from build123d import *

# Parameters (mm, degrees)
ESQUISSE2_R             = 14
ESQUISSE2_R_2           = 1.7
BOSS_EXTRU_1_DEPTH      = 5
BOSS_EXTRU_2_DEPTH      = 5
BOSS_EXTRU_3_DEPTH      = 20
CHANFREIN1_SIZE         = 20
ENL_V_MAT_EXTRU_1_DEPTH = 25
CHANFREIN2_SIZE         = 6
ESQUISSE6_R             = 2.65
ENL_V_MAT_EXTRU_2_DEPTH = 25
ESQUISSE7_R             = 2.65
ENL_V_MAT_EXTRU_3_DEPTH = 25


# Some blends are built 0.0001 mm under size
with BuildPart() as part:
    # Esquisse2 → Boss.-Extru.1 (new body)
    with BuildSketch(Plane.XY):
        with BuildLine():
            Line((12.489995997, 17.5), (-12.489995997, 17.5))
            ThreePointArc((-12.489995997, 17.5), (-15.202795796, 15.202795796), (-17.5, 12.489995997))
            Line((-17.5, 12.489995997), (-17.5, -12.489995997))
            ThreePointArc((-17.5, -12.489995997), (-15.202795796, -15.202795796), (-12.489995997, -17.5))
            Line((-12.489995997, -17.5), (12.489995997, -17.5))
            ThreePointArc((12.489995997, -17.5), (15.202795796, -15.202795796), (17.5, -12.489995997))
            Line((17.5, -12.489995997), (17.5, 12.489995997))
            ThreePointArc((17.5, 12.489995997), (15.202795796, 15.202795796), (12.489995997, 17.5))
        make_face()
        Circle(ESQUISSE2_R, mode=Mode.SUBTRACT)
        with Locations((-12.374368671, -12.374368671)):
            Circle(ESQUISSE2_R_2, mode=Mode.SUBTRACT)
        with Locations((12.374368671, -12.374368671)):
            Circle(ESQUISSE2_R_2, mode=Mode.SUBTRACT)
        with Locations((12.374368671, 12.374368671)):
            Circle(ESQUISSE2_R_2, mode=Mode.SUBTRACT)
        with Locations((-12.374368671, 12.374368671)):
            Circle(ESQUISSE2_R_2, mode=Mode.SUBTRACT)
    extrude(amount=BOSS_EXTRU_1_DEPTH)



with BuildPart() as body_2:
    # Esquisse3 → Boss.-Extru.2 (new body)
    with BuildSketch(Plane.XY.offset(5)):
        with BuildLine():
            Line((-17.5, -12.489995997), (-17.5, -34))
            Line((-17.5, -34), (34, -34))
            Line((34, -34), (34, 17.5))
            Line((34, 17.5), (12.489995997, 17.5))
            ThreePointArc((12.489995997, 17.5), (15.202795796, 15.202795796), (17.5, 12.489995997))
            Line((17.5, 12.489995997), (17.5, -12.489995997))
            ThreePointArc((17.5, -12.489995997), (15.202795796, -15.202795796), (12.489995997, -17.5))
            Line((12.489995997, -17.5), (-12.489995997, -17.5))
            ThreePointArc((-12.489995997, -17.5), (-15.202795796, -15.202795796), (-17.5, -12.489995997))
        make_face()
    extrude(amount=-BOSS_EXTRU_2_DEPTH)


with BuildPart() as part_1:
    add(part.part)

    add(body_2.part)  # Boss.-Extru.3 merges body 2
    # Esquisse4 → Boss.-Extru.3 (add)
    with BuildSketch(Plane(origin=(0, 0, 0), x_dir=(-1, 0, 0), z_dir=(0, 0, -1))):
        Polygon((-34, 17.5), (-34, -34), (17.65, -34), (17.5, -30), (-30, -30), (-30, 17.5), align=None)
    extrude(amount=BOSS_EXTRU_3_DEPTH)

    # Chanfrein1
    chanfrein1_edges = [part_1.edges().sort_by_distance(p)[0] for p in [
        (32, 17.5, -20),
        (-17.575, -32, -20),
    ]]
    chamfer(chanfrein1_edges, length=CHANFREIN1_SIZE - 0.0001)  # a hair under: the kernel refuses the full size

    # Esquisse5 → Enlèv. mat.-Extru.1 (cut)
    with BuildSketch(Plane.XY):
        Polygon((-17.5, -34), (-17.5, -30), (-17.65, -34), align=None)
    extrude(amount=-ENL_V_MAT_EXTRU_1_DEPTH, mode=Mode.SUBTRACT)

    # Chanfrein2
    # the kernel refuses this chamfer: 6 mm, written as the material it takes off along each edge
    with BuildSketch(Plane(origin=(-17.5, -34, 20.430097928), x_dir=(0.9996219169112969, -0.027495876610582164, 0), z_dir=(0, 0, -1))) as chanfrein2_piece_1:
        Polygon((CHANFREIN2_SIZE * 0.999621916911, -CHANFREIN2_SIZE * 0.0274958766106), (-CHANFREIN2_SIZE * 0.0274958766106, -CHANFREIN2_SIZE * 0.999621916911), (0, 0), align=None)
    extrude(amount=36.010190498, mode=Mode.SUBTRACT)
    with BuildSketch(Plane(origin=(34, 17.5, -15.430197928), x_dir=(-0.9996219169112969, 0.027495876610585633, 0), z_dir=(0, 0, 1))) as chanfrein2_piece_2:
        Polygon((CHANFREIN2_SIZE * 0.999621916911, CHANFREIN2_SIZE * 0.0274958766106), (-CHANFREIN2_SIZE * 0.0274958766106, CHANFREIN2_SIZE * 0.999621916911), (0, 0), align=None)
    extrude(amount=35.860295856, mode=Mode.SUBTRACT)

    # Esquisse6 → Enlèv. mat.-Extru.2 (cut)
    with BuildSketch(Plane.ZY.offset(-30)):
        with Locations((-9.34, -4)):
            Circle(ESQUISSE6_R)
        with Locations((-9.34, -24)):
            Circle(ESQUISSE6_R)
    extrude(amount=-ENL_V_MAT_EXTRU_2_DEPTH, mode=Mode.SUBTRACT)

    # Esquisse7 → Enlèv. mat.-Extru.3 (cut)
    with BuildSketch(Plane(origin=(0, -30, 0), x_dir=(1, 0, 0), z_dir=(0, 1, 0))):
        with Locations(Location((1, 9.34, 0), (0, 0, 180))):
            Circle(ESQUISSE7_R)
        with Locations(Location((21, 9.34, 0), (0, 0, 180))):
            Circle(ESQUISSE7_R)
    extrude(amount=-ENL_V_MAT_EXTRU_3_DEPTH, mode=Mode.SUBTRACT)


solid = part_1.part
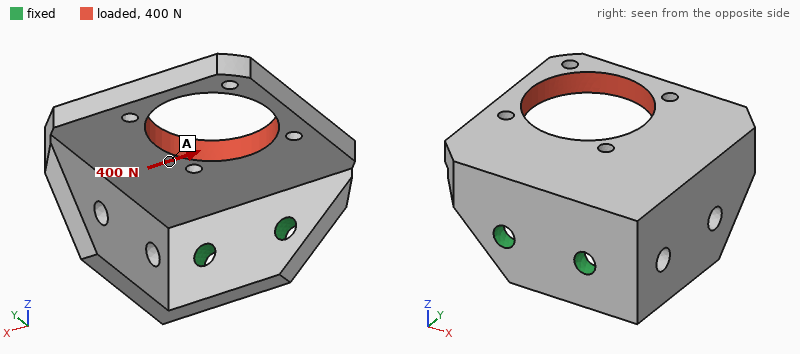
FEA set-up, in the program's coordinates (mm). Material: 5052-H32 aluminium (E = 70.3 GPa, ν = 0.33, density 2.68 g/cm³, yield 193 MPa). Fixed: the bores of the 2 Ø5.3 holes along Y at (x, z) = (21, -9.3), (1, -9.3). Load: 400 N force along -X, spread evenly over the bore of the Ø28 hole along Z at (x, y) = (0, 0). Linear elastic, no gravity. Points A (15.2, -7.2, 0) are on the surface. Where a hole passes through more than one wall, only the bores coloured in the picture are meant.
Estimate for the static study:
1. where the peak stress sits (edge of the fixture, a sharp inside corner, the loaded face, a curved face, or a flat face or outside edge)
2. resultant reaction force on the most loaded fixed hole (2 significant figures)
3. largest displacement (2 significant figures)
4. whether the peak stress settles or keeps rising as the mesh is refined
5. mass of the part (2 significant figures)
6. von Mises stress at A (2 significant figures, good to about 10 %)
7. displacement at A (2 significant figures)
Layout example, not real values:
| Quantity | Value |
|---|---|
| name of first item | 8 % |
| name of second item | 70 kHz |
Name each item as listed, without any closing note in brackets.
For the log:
| Quantity | Value |
|---|---|
| where the peak stress sits | edge of the fixture |
| resultant reaction force on the most loaded fixed hole | 550 N |
| largest displacement | 85 µm |
| whether the peak stress settles or keeps rising as the mesh is refined | keeps rising |
| mass of the part | 42 g |
| von Mises stress at A | 9.3 MPa |
| displacement at A | 35 µm |
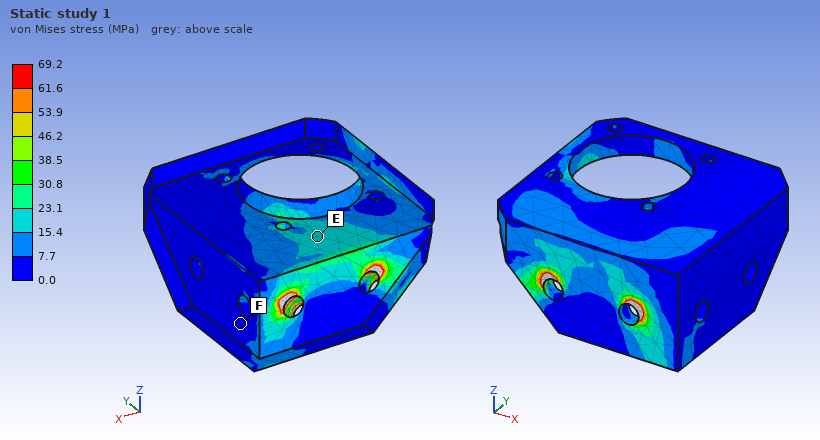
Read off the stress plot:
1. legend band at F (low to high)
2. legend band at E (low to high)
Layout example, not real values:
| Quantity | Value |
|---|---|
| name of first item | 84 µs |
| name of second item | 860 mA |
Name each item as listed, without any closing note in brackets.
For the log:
| Quantity | Value |
|---|---|
| legend band at F | 0.0 to 7.7 MPa |
| legend band at E | 15.4 to 23.1 MPa |
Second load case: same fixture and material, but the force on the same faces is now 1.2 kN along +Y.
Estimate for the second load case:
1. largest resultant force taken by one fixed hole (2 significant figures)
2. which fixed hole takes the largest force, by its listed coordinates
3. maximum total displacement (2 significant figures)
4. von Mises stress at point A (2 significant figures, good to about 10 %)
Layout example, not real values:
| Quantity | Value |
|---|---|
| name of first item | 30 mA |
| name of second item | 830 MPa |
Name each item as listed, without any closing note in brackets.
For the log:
| Quantity | Value |
|---|---|
| largest resultant force taken by one fixed hole | 1.1 kN |
| which fixed hole takes the largest force, by its listed coordinates | (1, -9.3) |
| maximum total displacement | 0.19 mm |
| von Mises stress at point A | 19 MPa |
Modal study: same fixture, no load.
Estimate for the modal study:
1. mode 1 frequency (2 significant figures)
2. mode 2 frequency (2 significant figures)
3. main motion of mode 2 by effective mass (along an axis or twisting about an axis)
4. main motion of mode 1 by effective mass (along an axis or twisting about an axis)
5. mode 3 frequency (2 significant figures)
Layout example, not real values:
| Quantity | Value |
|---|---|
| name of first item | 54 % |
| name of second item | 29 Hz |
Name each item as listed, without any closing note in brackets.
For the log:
| Quantity | Value |
|---|---|
| mode 1 frequency | 1600 Hz |
| mode 2 frequency | 2600 Hz |
| main motion of mode 2 by effective mass | along X |
| main motion of mode 1 by effective mass | along Z |
| mode 3 frequency | 4100 Hz |
